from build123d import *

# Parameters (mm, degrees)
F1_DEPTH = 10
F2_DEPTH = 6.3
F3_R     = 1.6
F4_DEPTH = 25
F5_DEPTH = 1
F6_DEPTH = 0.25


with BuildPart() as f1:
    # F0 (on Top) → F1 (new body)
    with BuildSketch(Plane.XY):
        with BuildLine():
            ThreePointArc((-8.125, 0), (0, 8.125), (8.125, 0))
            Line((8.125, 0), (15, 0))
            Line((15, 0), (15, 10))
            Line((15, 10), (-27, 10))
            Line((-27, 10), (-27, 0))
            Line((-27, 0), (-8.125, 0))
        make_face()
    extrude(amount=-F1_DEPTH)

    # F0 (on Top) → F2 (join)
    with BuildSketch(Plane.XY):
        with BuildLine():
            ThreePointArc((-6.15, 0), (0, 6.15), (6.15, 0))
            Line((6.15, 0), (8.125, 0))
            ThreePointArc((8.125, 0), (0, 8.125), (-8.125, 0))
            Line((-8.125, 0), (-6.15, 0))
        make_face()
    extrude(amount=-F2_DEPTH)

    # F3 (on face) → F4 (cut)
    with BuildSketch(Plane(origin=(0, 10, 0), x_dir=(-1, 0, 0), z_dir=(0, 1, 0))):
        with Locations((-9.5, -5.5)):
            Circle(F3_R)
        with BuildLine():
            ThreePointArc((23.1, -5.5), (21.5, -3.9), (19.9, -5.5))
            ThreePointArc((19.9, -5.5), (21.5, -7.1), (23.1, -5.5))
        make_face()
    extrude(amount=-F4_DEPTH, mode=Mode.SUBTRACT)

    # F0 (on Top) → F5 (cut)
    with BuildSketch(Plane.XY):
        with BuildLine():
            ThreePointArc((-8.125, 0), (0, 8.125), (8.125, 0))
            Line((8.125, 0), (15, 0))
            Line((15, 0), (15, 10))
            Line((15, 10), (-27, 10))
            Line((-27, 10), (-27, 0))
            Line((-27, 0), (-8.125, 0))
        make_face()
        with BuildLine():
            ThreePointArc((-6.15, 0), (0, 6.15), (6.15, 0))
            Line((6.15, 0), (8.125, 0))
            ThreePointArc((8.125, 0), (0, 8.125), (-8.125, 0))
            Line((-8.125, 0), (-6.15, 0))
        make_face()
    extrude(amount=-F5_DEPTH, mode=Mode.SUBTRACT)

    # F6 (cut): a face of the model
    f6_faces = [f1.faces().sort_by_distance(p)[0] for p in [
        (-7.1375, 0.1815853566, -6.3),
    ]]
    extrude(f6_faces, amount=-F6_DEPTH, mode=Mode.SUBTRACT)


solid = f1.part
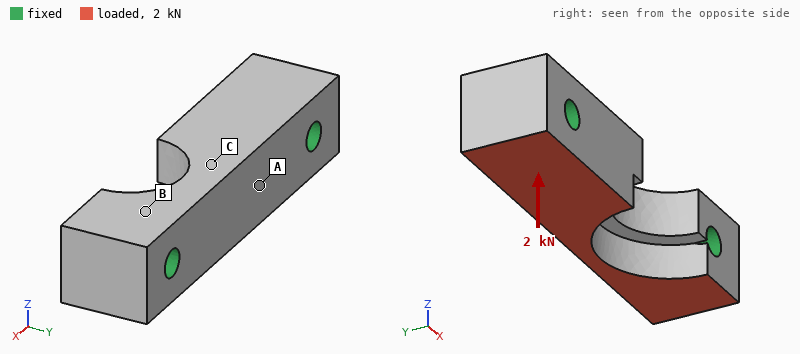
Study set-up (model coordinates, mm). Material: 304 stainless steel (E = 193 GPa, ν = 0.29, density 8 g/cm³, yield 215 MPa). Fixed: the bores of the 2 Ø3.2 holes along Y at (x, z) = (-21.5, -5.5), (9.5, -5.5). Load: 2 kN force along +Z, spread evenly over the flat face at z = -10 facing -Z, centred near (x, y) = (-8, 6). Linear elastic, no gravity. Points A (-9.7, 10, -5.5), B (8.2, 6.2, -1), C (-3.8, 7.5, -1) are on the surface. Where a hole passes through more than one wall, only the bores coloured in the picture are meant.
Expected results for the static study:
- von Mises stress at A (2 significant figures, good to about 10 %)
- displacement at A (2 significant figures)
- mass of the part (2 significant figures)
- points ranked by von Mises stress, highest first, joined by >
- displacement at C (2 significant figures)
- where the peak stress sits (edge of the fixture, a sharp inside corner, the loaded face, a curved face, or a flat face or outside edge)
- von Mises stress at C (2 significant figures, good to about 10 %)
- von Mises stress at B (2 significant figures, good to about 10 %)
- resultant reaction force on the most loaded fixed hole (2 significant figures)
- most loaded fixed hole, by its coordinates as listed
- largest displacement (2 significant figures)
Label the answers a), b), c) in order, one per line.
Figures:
a) 6.6 MPa
b) 2.5 µm
c) 23 g
d) C > B > A
e) 2.7 µm
f) edge of the fixture
g) 27 MPa
h) 17 MPa
i) 1.2 kN
j) (-21.5, -5.5)
k) 3.3 µm
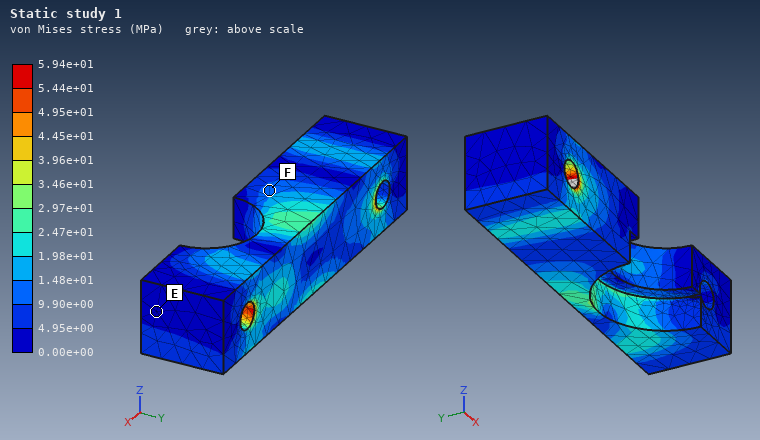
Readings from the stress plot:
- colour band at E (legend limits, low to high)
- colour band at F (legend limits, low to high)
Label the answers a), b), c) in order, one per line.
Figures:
a) 0.00e+00 to 4.95e+00 MPa
b) 9.90e+00 to 1.48e+01 MPa
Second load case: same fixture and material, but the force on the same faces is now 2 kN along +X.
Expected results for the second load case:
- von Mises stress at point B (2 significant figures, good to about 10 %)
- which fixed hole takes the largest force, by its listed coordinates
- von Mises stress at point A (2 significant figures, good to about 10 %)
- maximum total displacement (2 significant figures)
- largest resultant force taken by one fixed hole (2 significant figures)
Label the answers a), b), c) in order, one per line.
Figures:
a) 9.5 MPa
b) (-21.5, -5.5)
c) 5.5 MPa
d) 2.1 µm
e) 1.3 kN
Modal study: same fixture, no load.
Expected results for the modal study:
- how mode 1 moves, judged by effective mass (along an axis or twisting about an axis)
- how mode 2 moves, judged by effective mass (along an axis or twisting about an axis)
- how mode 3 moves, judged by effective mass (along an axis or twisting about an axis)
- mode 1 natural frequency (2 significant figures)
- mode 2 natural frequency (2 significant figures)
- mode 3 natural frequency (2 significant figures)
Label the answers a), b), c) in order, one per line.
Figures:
a) along Z
b) along Y
c) twisting about X
d) 28 kHz
e) 31 kHz
f) 45 kHz
